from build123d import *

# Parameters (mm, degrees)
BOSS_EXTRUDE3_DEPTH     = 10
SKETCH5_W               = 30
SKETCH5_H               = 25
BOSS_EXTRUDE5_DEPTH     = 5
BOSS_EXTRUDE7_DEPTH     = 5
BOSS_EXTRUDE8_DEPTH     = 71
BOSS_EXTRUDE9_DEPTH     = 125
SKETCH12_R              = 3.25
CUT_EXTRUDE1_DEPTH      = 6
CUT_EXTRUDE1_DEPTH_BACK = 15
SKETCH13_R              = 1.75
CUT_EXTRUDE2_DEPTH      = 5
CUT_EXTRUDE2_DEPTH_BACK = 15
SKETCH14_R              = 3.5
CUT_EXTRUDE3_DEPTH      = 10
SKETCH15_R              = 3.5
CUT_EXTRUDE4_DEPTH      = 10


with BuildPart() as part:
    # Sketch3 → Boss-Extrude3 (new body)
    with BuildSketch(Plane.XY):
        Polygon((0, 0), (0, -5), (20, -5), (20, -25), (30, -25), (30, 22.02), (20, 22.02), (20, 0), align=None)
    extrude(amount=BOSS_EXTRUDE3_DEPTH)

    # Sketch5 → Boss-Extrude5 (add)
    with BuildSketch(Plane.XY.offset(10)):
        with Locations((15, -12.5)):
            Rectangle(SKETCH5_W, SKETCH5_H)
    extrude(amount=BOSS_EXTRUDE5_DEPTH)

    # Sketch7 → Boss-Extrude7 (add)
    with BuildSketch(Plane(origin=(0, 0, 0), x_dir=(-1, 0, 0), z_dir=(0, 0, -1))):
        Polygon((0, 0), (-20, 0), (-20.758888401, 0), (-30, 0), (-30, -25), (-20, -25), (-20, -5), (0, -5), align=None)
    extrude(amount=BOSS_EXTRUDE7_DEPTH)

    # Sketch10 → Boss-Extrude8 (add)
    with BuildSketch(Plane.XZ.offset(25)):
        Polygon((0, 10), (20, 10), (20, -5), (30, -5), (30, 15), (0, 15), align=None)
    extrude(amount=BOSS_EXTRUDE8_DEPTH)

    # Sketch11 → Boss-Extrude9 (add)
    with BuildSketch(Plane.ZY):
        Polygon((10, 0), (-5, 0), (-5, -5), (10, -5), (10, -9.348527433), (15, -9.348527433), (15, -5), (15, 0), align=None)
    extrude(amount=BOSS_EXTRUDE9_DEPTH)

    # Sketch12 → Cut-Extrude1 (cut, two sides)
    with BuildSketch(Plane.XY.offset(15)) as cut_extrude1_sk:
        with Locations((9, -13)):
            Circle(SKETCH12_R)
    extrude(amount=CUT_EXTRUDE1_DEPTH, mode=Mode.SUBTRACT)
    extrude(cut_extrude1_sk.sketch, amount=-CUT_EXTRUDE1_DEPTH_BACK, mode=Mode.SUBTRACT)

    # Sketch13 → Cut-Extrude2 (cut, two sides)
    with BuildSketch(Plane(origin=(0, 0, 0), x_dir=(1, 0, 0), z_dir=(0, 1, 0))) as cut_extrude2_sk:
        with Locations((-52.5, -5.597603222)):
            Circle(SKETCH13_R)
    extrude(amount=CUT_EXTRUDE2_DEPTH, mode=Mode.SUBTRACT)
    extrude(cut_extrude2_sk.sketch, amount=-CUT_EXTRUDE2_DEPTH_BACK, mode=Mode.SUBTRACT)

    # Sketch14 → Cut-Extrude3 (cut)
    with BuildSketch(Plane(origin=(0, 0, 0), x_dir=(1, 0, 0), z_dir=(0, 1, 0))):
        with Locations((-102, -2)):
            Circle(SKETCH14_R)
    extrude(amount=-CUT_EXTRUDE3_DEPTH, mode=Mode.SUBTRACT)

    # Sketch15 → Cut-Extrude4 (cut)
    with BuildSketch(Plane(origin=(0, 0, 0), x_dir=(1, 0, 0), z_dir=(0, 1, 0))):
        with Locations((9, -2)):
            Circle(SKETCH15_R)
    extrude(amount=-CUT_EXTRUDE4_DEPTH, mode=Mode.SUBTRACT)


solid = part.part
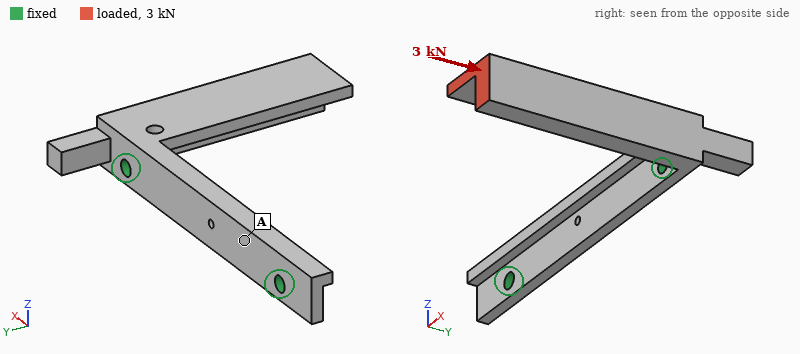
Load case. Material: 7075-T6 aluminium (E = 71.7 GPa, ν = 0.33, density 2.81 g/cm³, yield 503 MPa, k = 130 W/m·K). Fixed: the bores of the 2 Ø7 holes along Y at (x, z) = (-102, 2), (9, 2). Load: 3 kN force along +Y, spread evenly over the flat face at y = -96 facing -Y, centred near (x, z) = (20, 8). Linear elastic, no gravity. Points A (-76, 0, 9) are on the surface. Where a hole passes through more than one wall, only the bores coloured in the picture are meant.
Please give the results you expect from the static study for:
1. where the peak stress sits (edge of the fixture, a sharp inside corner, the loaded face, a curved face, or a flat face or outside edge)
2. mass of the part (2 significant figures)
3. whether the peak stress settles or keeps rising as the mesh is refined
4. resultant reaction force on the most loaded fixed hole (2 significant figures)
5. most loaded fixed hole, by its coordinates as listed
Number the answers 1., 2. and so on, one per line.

1. edge of the fixture
2. 130 g
3. keeps rising
4. 3.1 kN
5. (9, 2)
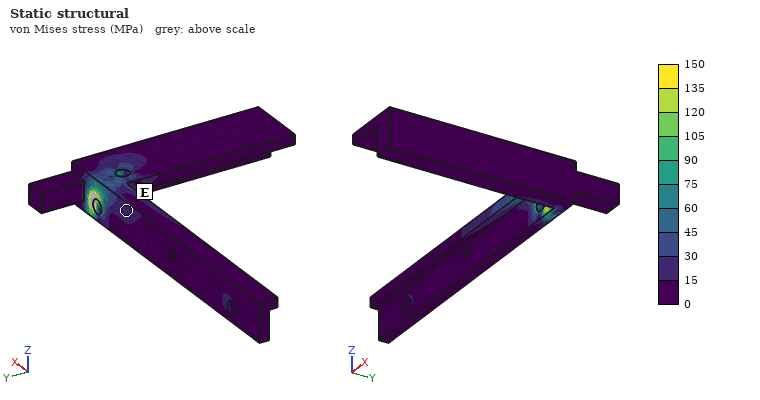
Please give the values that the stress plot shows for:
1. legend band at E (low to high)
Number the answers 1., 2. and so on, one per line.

1. 15 to 30 MPa
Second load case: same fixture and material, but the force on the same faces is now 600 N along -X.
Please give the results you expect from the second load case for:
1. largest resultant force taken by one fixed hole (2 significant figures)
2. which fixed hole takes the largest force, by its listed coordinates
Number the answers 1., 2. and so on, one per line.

1. 570 N
2. (-102, 2)
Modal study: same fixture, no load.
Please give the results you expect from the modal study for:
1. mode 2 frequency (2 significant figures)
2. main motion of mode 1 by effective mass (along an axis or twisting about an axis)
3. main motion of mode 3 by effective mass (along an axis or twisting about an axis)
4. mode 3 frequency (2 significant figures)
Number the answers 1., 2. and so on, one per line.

1. 860 Hz
2. along Z
3. along Y
4. 2900 Hz
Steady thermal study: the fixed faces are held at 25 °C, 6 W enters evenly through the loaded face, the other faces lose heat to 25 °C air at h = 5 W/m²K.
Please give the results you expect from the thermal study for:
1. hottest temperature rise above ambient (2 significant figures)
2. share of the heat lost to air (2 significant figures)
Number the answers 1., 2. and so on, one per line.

1. 17 K
2. 8.3 %
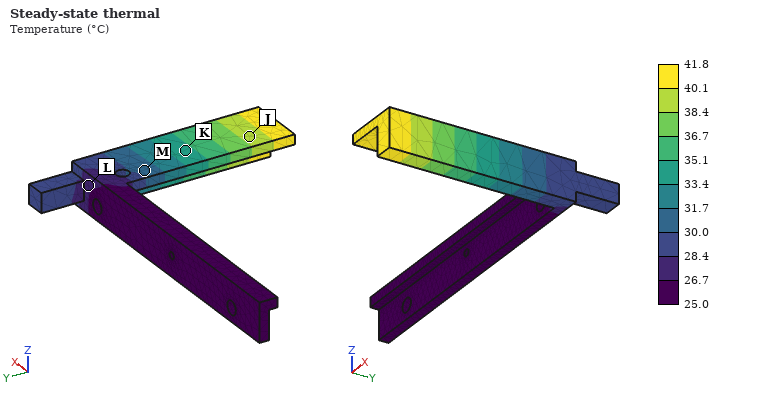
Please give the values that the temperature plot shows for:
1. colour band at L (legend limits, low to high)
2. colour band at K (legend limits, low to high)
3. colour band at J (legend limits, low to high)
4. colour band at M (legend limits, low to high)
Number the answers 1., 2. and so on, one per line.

1. 26.7 to 28.4 °C
2. 33.4 to 35.1 °C
3. 38.4 to 40.1 °C
4. 30.0 to 31.7 °C
